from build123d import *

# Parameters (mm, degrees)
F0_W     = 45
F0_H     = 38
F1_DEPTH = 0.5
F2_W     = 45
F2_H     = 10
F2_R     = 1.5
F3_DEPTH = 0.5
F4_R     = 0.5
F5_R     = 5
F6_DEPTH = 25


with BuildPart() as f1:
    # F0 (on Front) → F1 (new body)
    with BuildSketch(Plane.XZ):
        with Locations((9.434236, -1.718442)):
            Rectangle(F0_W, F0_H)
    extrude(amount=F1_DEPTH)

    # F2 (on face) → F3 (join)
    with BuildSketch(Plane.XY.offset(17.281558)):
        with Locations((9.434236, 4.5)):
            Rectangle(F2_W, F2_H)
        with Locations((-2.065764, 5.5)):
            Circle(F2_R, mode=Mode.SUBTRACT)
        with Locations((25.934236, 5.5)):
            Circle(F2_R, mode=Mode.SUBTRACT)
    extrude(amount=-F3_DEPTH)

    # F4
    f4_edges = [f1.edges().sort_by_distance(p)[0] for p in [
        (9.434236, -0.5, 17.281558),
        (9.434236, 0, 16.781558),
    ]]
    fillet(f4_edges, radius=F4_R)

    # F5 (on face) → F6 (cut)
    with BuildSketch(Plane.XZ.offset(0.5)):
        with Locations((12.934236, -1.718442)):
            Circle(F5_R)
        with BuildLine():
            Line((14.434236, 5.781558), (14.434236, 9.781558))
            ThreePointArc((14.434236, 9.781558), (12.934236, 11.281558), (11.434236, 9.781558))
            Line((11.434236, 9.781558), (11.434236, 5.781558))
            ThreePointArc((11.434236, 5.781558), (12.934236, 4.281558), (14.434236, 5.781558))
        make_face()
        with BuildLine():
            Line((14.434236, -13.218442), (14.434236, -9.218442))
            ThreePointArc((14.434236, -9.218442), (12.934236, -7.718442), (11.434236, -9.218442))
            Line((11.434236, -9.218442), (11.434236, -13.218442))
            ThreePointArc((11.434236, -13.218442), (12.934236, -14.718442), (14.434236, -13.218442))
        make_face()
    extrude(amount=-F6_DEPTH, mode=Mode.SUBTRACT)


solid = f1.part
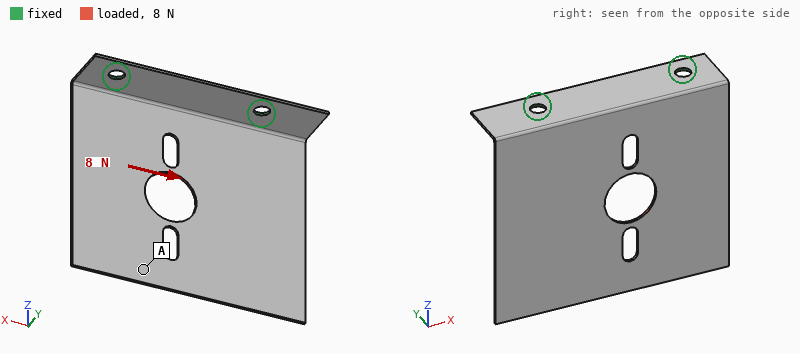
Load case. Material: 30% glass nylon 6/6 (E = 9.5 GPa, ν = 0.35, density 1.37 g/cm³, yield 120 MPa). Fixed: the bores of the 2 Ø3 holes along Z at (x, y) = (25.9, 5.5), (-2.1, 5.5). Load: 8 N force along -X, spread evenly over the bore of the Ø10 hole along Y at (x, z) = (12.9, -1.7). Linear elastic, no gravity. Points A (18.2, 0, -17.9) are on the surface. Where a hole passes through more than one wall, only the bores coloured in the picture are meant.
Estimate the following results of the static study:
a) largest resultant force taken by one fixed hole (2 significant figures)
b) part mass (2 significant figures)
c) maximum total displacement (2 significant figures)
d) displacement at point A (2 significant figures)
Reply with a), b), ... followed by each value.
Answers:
a) 6.7 N
b) 1.4 g
c) 0.67 mm
d) 0.31 mm
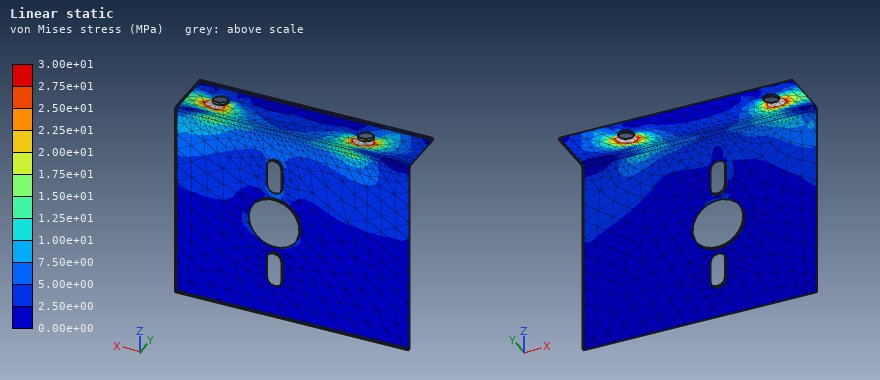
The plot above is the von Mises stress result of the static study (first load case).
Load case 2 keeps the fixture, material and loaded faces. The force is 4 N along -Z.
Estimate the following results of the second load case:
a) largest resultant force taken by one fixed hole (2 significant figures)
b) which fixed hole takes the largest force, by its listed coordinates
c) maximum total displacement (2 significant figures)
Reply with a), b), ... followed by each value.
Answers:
a) 2.1 N
b) (25.9, 5.5)
c) 0.57 mm
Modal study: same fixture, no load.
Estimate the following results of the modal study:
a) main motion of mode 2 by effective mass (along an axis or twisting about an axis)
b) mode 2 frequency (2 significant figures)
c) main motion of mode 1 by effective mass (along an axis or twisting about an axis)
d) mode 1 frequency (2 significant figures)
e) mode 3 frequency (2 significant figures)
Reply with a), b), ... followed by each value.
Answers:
a) twisting about Z
b) 280 Hz
c) along Y
d) 120 Hz
e) 740 Hz
